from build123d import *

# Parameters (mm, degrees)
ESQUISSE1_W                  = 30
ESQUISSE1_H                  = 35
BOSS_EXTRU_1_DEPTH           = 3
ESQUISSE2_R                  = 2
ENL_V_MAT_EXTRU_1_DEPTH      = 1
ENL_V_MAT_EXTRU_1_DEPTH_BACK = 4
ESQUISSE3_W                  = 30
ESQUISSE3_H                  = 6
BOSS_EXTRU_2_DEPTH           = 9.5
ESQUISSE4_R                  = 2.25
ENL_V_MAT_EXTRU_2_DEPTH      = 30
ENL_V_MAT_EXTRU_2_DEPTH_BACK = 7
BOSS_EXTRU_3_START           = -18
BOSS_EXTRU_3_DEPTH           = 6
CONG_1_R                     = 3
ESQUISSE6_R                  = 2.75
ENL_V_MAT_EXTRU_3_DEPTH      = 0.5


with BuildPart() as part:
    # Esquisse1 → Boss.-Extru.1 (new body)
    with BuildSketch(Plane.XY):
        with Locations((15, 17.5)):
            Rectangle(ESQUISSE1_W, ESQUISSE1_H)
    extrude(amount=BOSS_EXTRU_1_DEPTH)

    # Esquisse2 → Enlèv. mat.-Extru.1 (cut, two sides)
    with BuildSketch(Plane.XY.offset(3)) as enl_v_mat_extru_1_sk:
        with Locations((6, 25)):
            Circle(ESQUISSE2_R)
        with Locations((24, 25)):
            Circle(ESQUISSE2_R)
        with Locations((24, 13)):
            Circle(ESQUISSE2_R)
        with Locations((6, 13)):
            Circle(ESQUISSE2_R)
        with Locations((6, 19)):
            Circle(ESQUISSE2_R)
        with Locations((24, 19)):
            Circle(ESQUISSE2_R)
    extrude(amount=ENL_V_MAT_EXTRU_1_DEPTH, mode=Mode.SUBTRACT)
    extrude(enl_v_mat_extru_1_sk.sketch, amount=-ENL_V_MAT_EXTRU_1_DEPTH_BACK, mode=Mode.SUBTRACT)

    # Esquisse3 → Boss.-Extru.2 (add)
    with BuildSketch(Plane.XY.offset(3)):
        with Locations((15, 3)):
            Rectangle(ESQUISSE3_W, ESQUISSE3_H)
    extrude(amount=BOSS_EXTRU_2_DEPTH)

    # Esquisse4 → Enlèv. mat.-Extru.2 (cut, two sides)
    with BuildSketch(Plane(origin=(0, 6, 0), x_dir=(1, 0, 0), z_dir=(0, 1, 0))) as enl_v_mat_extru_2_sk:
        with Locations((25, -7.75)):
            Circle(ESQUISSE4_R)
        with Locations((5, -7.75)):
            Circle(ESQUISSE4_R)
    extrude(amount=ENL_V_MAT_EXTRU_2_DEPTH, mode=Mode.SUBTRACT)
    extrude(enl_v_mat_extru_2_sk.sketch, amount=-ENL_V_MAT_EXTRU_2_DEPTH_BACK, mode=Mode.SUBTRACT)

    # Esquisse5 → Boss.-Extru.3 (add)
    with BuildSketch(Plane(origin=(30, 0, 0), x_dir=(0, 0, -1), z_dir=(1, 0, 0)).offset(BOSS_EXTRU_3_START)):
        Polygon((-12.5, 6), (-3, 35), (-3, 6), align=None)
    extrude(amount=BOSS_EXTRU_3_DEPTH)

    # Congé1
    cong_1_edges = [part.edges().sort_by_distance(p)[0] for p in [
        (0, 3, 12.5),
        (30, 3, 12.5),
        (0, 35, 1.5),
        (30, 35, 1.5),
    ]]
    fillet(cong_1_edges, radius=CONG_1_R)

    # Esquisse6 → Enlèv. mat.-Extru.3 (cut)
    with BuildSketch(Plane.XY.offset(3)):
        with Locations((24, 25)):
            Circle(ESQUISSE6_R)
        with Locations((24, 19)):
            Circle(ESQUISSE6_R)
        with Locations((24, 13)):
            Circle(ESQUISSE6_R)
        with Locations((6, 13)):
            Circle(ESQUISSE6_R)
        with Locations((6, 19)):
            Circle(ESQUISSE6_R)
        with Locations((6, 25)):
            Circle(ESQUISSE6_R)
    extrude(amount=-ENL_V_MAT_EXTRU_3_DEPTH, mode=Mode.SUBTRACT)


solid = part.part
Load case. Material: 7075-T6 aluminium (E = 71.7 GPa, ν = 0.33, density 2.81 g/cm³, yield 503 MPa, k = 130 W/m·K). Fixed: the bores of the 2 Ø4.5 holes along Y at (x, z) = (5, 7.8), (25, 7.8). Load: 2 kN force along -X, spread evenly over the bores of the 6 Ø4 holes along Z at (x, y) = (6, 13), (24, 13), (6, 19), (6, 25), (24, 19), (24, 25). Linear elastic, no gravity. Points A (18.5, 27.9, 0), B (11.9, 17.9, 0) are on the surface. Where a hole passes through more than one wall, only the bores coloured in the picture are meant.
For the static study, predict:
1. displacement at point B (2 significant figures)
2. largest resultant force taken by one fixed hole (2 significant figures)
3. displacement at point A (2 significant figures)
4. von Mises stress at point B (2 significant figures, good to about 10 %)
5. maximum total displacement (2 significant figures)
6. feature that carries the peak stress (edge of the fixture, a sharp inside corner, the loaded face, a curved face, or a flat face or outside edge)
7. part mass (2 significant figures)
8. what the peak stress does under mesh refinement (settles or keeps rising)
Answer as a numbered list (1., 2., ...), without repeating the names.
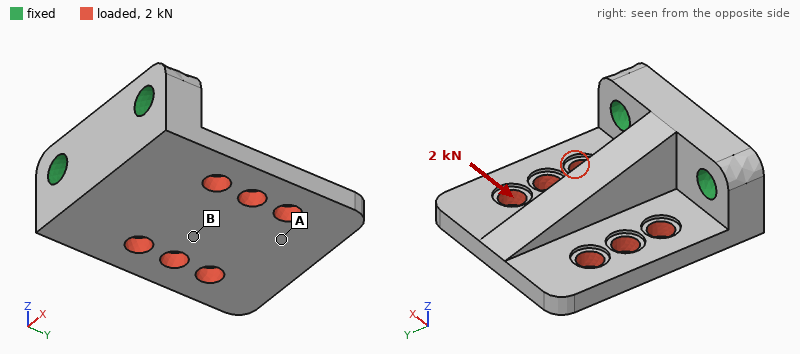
1. 27 µm
2. 1.9 kN
3. 45 µm
4. 43 MPa
5. 57 µm
6. edge of the fixture
7. 15 g
8. keeps rising
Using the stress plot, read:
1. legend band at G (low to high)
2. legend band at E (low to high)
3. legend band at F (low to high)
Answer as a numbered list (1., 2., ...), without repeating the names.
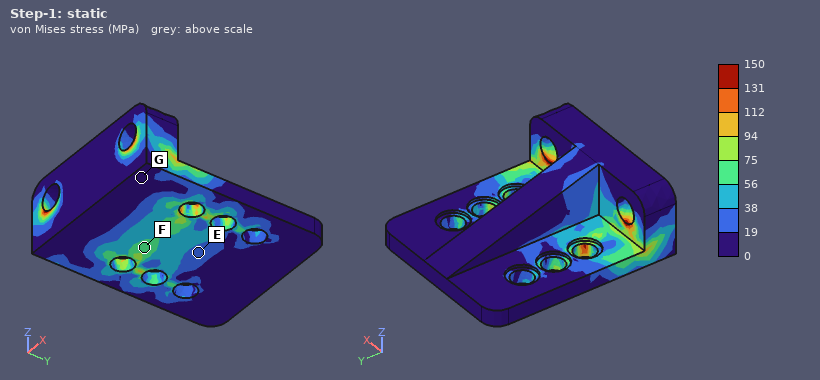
1. 0 to 19 MPa
2. 19 to 38 MPa
3. 56 to 75 MPa
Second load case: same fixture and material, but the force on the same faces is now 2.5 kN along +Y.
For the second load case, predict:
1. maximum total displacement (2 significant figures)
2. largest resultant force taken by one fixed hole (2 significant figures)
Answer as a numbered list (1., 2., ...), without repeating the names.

1. 61 µm
2. 1.3 kN
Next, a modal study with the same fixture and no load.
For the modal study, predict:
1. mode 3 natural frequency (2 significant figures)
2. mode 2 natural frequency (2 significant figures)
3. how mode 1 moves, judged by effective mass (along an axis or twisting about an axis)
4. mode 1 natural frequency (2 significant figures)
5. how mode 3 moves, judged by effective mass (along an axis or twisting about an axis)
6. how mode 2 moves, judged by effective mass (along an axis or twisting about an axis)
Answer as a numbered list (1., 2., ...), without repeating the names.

1. 12 kHz
2. 8400 Hz
3. along Z
4. 5900 Hz
5. along X
6. twisting about Y
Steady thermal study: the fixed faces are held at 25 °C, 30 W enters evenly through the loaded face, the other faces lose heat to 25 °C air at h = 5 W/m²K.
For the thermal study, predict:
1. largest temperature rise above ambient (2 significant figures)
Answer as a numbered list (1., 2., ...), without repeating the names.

1. 40 K
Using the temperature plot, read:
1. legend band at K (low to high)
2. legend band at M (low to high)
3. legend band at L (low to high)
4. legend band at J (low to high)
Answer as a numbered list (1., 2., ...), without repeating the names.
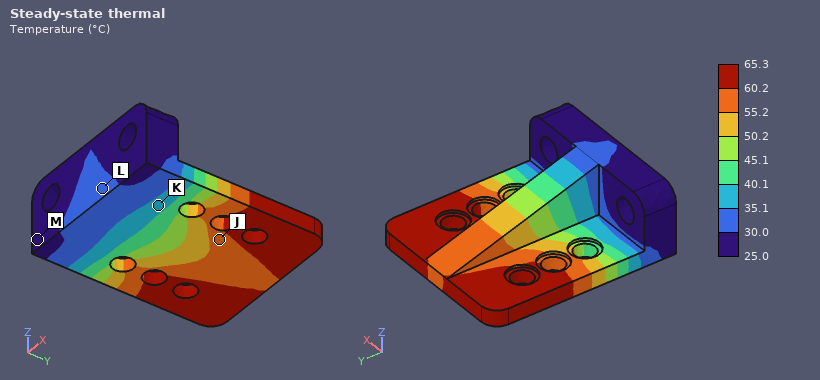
1. 35.1 to 40.1 °C
2. 25.0 to 30.0 °C
3. 30.0 to 35.1 °C
4. 55.2 to 60.2 °C
